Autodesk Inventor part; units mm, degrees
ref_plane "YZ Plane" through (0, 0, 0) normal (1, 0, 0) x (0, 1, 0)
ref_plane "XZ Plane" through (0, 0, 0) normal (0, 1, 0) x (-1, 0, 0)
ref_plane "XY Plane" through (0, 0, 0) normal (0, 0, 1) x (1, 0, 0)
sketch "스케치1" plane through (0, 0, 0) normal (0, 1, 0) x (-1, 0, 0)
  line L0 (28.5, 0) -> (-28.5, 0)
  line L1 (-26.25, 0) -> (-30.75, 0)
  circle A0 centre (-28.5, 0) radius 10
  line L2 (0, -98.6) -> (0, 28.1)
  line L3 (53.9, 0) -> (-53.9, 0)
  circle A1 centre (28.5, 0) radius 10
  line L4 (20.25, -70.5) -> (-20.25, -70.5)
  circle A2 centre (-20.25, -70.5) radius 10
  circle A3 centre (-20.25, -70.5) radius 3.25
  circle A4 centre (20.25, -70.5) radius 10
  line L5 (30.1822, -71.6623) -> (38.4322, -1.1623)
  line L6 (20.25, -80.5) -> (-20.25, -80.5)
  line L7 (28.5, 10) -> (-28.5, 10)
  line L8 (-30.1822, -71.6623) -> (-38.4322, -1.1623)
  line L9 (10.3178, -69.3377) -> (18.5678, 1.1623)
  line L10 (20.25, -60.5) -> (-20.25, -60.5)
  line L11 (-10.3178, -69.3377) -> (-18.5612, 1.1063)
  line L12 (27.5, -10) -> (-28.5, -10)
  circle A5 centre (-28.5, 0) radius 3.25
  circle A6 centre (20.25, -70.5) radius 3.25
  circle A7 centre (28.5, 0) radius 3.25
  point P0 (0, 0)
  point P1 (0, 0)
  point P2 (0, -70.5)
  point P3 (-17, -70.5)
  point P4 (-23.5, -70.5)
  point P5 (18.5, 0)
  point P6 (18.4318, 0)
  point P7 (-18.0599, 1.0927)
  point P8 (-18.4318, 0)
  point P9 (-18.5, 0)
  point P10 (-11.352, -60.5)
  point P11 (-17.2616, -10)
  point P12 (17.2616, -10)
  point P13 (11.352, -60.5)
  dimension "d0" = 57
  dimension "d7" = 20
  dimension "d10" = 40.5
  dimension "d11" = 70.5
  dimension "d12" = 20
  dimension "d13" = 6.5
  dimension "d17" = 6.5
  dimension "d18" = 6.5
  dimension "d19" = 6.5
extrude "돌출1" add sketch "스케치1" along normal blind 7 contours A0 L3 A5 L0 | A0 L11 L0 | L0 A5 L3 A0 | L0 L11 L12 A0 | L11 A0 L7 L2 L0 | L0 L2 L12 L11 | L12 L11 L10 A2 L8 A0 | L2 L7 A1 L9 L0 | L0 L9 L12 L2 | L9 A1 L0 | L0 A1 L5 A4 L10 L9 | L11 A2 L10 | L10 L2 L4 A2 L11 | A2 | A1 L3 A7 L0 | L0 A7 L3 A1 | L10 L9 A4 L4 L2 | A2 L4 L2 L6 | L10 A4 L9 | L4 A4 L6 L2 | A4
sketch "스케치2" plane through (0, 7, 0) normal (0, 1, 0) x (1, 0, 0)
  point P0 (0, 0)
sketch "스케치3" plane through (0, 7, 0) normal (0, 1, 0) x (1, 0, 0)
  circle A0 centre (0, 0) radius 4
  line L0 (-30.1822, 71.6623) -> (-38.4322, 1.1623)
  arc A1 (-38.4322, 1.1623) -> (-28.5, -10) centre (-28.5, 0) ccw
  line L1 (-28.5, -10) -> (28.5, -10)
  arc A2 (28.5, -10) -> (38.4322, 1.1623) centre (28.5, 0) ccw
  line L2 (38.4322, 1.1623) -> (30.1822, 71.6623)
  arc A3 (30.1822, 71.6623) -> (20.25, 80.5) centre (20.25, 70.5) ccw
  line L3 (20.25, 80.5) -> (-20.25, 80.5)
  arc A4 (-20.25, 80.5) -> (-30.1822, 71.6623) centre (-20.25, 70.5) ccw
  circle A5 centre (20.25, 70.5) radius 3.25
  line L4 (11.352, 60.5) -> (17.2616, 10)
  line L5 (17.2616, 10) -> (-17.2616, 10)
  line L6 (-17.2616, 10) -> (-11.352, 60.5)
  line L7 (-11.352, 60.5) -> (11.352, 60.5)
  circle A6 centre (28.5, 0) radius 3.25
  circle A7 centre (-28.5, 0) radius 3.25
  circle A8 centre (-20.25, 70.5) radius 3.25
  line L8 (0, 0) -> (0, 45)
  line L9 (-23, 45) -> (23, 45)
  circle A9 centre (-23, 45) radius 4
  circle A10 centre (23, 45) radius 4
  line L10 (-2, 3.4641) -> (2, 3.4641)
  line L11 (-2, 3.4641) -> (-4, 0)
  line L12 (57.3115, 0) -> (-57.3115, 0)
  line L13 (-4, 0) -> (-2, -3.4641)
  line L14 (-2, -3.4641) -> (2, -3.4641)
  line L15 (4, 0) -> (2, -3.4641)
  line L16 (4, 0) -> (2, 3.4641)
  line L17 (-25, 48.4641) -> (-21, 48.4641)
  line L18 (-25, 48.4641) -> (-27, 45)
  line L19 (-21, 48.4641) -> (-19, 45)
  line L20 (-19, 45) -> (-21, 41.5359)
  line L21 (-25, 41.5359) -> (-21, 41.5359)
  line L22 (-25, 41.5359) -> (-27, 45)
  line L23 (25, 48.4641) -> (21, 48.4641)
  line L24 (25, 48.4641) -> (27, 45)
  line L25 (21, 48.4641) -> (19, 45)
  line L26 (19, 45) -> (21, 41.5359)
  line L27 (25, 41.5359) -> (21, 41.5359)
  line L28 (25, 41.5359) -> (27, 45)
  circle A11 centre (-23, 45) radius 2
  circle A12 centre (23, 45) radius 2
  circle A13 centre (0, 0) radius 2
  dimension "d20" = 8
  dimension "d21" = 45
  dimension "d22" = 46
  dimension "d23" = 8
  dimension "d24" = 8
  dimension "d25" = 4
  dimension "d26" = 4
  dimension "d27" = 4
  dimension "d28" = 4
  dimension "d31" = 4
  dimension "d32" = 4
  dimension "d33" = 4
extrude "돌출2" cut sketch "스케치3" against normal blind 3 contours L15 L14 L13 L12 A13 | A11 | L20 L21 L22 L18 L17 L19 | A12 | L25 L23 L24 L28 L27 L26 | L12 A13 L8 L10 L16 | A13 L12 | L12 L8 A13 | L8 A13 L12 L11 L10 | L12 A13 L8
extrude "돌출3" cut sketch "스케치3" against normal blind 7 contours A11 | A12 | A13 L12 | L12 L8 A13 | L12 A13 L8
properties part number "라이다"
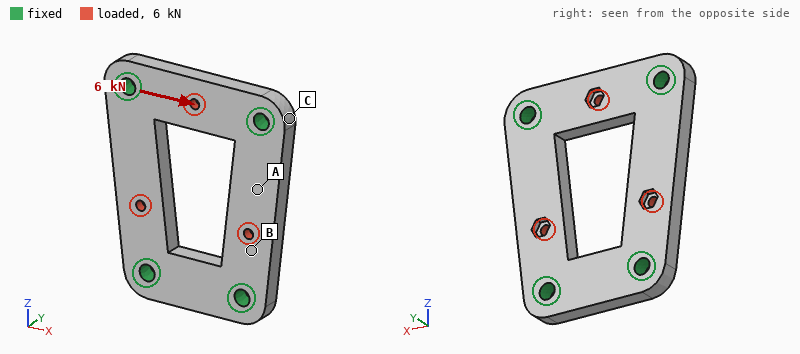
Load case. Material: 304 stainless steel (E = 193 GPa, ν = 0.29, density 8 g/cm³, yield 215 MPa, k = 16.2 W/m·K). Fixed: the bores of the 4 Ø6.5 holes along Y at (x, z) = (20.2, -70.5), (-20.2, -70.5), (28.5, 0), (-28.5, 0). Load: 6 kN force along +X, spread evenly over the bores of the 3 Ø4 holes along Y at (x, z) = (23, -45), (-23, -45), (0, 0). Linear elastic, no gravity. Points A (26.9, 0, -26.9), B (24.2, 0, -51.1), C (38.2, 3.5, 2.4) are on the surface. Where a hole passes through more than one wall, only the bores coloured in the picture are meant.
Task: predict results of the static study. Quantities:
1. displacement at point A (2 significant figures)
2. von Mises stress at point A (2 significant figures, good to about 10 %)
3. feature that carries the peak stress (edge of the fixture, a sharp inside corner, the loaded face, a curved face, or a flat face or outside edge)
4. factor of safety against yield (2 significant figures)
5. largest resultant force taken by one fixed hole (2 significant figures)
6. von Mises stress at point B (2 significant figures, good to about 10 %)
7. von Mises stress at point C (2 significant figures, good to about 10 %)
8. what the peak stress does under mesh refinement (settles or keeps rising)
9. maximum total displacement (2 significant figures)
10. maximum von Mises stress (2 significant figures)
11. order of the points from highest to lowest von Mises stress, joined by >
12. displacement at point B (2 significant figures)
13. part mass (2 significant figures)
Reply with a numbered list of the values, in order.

1. 5.3 µm
2. 17 MPa
3. the loaded face
4. 2.9
5. 1.6 kN
6. 32 MPa
7. 7.1 MPa
8. settles
9. 8.2 µm
10. 73 MPa
11. B > A > C
12. 5.8 µm
13. 250 g
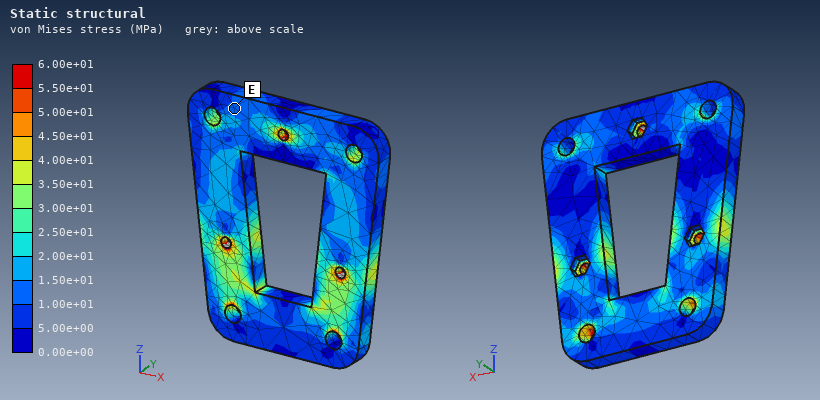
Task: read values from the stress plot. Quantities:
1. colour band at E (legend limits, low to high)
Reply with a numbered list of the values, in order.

1. 1.00e+01 to 1.50e+01 MPa
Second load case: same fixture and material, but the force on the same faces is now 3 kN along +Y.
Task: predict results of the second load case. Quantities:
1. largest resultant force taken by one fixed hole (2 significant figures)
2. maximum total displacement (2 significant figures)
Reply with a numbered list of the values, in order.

1. 800 N
2. 16 µm
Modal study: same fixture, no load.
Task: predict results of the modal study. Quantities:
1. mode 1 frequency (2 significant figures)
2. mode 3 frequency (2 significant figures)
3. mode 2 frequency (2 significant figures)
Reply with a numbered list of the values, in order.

1. 7200 Hz
2. 11 kHz
3. 7300 Hz
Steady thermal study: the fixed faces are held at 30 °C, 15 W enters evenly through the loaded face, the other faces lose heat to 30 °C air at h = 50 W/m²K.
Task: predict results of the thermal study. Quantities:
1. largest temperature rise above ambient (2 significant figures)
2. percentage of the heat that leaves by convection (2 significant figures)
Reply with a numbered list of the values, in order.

1. 35 K
2. 41 %
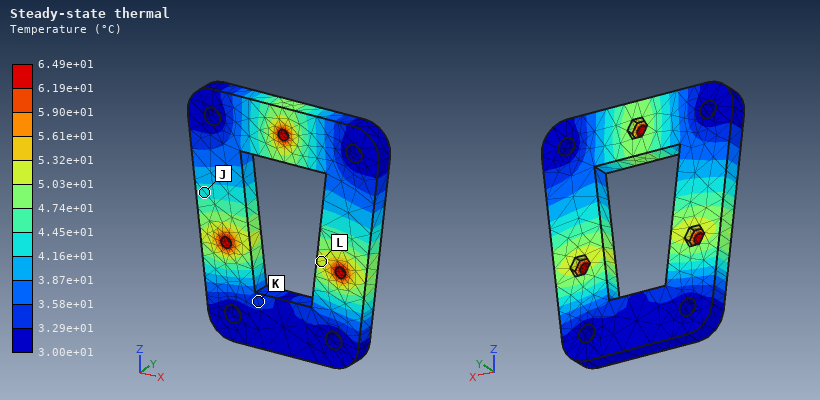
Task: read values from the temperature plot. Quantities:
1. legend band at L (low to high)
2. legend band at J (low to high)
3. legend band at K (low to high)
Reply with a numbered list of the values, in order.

1. 5.03e+01 to 5.32e+01 °C
2. 4.16e+01 to 4.45e+01 °C
3. 3.29e+01 to 3.58e+01 °C
